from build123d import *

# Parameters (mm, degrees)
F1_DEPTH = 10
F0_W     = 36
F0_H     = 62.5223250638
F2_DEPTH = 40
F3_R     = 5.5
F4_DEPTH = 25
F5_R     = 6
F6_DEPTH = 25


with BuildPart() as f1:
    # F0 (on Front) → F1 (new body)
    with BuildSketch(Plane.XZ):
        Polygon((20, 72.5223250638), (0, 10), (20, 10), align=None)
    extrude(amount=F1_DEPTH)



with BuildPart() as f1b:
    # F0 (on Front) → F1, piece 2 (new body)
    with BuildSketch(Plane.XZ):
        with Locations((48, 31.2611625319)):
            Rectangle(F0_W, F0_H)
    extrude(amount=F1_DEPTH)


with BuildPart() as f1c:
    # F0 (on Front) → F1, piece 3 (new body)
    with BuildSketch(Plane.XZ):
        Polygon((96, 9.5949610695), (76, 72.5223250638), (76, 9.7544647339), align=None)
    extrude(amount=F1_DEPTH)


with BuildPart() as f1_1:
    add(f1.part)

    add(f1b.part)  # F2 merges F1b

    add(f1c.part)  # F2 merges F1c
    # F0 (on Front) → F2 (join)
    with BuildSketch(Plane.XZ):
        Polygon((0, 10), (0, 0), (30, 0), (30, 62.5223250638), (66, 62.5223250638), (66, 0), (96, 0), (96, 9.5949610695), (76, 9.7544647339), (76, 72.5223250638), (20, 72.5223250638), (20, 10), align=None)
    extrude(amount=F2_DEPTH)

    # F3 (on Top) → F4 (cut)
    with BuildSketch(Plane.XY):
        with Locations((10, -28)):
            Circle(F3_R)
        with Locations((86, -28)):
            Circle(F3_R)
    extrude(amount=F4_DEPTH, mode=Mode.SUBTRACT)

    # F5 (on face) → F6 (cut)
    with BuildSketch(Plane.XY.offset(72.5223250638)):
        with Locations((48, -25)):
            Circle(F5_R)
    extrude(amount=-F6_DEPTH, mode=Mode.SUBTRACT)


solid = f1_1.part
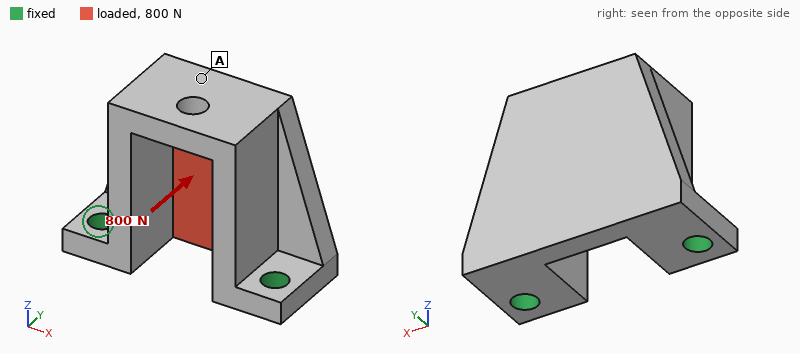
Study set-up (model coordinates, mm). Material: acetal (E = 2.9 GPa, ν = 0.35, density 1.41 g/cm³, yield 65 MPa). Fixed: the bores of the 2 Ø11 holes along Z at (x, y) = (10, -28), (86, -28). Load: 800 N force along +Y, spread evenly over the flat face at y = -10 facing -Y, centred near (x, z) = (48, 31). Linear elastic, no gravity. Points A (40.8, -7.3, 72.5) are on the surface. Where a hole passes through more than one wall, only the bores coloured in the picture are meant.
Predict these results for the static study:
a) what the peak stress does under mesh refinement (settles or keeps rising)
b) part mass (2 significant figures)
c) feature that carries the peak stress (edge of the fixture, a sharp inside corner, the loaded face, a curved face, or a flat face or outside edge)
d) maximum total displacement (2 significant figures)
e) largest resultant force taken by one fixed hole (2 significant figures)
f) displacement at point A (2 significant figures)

keeps rising
170 g
edge of the fixture
0.63 mm
450 N
0.61 mm
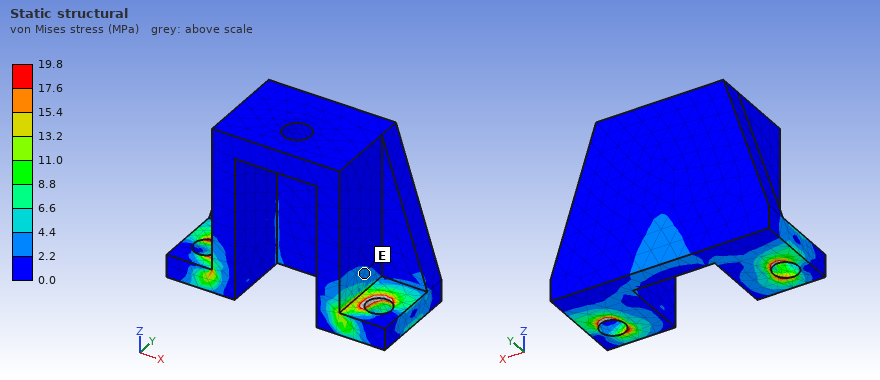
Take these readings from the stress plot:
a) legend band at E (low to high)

2.2 to 4.4 MPa
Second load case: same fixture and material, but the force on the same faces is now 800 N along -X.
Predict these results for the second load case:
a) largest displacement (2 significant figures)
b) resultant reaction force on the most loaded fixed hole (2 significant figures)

0.20 mm
500 N
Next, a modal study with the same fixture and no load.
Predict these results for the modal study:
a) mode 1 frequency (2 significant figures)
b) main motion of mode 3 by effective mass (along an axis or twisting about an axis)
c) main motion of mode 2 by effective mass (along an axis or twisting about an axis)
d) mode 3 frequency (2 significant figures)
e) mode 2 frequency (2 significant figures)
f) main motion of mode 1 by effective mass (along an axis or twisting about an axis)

470 Hz
along X
along X
1700 Hz
780 Hz
along Y
